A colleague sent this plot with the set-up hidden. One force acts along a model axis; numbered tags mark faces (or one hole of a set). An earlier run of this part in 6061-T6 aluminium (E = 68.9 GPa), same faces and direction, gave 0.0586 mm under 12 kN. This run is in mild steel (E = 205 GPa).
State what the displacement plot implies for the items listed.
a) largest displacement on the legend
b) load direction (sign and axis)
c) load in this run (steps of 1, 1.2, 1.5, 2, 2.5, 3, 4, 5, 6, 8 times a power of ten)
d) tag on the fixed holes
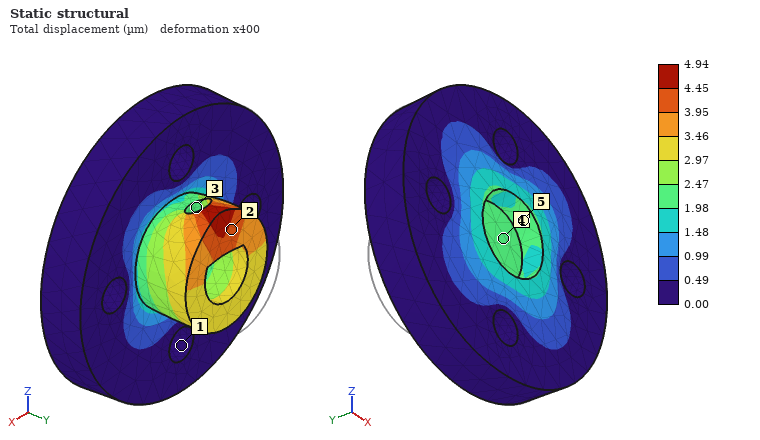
4.94 µm
-Y
3 kN
1
